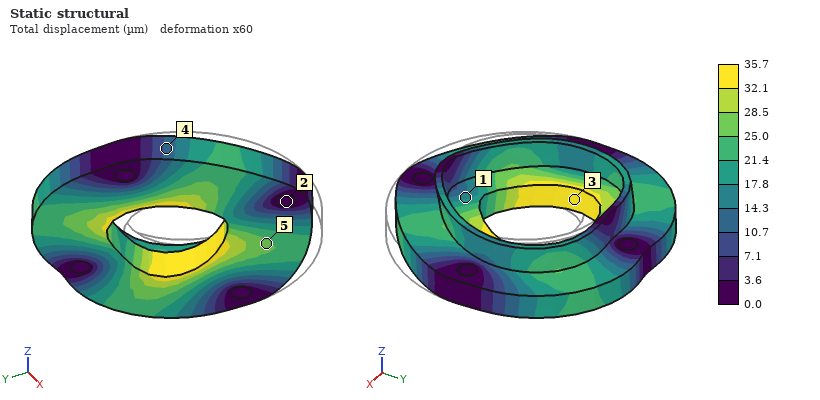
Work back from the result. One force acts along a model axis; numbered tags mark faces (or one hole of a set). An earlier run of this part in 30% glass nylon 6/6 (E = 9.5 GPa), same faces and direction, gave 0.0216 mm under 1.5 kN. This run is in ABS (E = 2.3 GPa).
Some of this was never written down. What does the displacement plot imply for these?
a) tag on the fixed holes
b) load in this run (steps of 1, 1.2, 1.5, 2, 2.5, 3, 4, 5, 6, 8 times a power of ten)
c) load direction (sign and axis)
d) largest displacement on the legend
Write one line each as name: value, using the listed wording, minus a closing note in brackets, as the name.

tag on the fixed holes: 2
load in this run: 600 N
load direction: +Y
largest displacement on the legend: 35.7 µm
